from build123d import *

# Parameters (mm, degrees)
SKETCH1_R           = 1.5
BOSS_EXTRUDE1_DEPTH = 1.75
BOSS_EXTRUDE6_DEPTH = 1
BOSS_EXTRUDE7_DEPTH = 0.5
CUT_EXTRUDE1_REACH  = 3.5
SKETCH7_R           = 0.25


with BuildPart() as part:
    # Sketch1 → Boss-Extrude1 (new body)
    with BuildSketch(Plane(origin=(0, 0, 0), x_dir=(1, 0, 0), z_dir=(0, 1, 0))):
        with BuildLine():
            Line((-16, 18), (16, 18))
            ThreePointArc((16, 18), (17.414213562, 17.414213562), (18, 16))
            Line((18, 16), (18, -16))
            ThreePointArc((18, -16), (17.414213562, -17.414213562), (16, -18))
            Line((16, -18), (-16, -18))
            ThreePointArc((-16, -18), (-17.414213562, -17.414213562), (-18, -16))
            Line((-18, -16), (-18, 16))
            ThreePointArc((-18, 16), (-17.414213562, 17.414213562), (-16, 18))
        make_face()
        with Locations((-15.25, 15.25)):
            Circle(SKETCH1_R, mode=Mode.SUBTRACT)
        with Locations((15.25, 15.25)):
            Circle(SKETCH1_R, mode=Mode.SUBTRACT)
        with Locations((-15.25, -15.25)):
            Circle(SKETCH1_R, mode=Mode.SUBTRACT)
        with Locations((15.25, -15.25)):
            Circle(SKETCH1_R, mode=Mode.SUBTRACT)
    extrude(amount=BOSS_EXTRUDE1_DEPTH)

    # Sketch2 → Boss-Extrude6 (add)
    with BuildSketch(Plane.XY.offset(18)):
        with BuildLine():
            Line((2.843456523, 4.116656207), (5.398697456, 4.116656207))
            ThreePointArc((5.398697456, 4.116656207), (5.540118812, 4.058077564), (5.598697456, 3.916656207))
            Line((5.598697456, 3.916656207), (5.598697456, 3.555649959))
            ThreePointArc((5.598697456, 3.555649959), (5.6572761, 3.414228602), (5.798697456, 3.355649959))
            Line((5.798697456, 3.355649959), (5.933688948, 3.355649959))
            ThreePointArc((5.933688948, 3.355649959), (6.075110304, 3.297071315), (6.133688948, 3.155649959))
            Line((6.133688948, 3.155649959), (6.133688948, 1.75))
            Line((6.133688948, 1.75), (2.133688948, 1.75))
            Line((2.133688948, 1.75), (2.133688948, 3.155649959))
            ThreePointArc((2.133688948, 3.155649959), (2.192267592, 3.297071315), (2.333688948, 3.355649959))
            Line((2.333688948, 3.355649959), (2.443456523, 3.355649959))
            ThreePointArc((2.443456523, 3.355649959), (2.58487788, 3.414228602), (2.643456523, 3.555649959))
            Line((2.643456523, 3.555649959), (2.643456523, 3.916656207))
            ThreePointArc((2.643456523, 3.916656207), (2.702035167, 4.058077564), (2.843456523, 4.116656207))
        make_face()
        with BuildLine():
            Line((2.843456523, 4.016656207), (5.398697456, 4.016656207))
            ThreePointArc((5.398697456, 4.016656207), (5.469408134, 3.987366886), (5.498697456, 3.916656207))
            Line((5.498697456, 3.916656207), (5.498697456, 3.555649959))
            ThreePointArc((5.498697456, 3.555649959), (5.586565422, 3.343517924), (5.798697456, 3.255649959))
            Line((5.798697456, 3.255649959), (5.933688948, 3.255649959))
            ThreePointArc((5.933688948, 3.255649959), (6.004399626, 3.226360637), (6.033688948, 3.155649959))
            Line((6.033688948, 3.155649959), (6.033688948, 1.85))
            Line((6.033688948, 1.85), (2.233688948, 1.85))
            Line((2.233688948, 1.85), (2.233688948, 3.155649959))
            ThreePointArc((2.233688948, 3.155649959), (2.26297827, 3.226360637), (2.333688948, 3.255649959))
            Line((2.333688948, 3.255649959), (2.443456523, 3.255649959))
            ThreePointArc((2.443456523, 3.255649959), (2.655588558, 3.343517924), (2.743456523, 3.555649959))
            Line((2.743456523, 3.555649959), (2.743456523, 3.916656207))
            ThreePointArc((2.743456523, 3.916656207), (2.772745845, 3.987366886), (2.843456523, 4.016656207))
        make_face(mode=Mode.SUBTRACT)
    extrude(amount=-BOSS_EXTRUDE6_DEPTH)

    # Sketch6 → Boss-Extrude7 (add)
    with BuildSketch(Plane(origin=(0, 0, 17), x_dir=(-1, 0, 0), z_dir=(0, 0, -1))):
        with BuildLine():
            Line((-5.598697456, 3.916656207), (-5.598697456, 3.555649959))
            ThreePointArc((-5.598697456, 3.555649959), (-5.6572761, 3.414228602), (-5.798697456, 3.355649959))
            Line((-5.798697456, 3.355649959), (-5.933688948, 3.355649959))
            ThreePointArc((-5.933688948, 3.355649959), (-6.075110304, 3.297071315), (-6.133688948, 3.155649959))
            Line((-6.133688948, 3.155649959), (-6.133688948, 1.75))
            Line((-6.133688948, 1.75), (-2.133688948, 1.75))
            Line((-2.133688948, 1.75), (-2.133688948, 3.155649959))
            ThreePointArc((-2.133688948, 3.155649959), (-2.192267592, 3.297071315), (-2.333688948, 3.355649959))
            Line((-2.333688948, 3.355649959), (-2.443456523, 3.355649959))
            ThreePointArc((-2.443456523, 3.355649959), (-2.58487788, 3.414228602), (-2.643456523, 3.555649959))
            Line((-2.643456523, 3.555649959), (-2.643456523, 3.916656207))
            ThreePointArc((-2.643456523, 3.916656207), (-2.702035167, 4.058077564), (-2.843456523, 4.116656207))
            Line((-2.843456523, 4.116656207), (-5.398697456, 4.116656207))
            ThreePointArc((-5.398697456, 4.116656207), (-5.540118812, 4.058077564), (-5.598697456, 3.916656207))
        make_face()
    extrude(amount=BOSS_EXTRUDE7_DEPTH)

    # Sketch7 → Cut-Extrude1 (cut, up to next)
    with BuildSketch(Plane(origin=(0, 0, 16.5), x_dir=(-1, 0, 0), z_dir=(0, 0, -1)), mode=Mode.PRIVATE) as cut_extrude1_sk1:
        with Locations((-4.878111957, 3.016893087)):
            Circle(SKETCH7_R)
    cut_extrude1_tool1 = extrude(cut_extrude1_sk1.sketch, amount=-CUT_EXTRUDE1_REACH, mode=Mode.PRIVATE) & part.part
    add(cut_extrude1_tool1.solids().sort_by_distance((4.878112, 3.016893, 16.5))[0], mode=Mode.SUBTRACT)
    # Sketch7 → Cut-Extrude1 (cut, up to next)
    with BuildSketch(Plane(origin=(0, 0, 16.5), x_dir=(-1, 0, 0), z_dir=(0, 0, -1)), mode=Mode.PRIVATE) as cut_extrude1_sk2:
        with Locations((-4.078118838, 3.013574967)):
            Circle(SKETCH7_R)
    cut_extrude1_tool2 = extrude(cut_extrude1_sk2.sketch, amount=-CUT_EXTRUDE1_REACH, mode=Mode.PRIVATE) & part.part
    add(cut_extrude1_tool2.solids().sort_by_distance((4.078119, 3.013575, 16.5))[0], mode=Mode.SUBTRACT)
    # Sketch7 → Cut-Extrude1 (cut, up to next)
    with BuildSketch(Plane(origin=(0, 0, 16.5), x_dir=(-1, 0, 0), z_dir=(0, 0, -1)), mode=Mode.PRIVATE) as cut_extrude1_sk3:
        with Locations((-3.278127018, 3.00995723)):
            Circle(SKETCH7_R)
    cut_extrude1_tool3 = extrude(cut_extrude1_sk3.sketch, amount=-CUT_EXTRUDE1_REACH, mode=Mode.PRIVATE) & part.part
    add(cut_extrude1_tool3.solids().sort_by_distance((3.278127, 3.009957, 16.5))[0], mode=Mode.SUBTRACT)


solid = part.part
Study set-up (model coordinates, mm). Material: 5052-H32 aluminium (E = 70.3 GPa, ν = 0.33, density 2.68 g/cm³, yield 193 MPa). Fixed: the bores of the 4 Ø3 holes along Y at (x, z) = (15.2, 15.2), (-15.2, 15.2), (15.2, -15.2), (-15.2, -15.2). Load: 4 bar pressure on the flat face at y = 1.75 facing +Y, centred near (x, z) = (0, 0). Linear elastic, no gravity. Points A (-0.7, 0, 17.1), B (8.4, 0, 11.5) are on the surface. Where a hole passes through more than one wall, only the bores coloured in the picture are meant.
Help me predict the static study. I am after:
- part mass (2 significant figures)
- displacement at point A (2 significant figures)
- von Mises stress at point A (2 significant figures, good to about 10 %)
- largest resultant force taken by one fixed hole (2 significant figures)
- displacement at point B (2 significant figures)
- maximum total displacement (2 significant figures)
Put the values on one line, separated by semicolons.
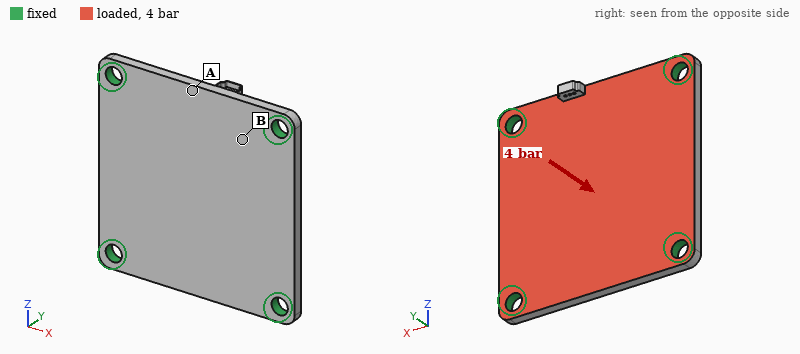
5.9 g; 28 µm; 37 MPa; 130 N; 26 µm; 64 µm
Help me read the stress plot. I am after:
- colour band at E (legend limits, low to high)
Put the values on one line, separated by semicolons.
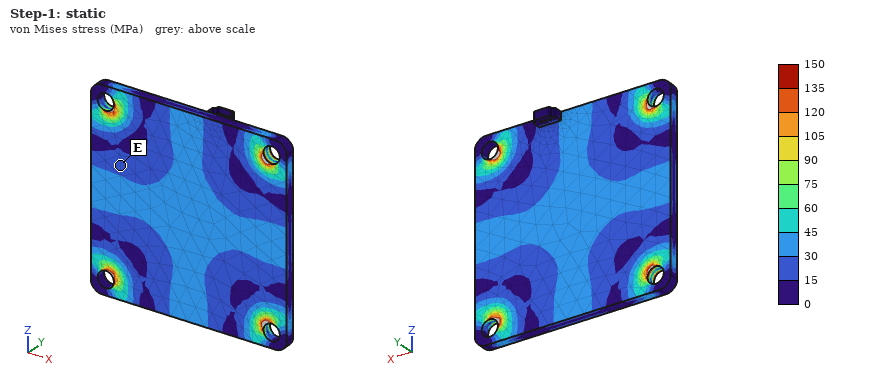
15 to 30 MPa
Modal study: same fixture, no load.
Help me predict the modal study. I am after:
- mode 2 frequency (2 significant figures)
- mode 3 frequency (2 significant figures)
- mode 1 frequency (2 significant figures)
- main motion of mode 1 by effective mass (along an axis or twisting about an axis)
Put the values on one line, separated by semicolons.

12 kHz; 12 kHz; 7100 Hz; along Y
